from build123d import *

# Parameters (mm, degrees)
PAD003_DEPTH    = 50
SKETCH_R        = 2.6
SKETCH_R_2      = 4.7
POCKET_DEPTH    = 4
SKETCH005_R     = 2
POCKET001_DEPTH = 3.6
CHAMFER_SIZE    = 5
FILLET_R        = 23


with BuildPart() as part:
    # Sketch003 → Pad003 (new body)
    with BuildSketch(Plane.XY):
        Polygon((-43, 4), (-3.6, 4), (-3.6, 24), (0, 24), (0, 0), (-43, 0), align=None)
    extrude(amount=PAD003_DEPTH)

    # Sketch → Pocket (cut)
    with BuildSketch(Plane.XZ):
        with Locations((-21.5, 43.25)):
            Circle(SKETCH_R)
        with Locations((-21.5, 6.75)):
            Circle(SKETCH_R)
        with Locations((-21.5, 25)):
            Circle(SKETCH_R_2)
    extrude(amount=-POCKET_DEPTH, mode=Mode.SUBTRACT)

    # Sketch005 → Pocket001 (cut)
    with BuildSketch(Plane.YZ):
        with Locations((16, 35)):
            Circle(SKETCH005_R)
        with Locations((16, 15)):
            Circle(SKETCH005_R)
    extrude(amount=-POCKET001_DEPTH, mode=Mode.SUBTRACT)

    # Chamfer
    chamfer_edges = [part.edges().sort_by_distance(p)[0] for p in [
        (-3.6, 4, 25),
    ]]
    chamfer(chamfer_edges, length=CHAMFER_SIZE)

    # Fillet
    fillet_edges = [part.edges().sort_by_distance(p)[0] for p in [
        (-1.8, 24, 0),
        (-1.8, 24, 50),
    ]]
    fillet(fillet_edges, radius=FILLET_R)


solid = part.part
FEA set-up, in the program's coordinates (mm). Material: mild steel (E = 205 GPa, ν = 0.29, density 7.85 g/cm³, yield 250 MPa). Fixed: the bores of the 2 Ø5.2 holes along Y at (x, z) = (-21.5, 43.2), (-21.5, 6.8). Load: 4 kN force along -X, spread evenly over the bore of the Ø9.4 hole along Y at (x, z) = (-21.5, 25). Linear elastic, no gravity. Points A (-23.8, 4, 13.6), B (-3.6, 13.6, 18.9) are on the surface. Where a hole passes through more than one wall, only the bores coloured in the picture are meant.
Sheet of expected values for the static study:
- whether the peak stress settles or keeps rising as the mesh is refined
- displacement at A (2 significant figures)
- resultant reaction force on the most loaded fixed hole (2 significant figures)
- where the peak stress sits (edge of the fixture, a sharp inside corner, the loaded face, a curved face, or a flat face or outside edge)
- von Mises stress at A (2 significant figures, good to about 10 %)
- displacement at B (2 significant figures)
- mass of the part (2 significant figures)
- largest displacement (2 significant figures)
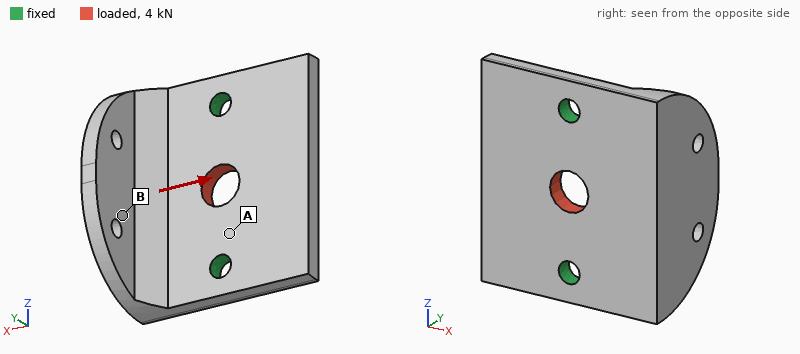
keeps rising
1.7 µm
2.0 kN
edge of the fixture
30 MPa
2.7 µm
90 g
4.1 µm
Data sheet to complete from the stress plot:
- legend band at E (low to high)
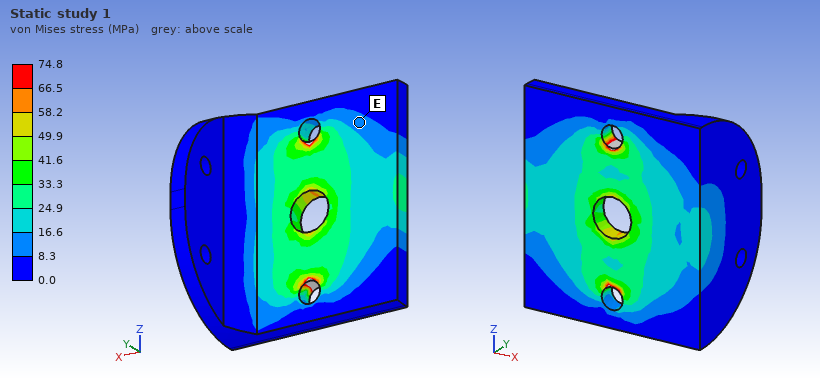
8.3 to 16.6 MPa
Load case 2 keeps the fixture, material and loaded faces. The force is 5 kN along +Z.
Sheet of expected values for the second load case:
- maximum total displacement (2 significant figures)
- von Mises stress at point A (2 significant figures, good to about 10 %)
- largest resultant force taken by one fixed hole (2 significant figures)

3.4 µm
48 MPa
2.5 kN
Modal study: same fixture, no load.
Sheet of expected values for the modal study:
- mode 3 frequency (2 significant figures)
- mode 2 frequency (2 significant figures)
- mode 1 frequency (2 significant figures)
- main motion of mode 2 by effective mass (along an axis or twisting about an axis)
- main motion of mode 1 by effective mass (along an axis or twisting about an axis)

7000 Hz
6500 Hz
3200 Hz
along Y
along Y
